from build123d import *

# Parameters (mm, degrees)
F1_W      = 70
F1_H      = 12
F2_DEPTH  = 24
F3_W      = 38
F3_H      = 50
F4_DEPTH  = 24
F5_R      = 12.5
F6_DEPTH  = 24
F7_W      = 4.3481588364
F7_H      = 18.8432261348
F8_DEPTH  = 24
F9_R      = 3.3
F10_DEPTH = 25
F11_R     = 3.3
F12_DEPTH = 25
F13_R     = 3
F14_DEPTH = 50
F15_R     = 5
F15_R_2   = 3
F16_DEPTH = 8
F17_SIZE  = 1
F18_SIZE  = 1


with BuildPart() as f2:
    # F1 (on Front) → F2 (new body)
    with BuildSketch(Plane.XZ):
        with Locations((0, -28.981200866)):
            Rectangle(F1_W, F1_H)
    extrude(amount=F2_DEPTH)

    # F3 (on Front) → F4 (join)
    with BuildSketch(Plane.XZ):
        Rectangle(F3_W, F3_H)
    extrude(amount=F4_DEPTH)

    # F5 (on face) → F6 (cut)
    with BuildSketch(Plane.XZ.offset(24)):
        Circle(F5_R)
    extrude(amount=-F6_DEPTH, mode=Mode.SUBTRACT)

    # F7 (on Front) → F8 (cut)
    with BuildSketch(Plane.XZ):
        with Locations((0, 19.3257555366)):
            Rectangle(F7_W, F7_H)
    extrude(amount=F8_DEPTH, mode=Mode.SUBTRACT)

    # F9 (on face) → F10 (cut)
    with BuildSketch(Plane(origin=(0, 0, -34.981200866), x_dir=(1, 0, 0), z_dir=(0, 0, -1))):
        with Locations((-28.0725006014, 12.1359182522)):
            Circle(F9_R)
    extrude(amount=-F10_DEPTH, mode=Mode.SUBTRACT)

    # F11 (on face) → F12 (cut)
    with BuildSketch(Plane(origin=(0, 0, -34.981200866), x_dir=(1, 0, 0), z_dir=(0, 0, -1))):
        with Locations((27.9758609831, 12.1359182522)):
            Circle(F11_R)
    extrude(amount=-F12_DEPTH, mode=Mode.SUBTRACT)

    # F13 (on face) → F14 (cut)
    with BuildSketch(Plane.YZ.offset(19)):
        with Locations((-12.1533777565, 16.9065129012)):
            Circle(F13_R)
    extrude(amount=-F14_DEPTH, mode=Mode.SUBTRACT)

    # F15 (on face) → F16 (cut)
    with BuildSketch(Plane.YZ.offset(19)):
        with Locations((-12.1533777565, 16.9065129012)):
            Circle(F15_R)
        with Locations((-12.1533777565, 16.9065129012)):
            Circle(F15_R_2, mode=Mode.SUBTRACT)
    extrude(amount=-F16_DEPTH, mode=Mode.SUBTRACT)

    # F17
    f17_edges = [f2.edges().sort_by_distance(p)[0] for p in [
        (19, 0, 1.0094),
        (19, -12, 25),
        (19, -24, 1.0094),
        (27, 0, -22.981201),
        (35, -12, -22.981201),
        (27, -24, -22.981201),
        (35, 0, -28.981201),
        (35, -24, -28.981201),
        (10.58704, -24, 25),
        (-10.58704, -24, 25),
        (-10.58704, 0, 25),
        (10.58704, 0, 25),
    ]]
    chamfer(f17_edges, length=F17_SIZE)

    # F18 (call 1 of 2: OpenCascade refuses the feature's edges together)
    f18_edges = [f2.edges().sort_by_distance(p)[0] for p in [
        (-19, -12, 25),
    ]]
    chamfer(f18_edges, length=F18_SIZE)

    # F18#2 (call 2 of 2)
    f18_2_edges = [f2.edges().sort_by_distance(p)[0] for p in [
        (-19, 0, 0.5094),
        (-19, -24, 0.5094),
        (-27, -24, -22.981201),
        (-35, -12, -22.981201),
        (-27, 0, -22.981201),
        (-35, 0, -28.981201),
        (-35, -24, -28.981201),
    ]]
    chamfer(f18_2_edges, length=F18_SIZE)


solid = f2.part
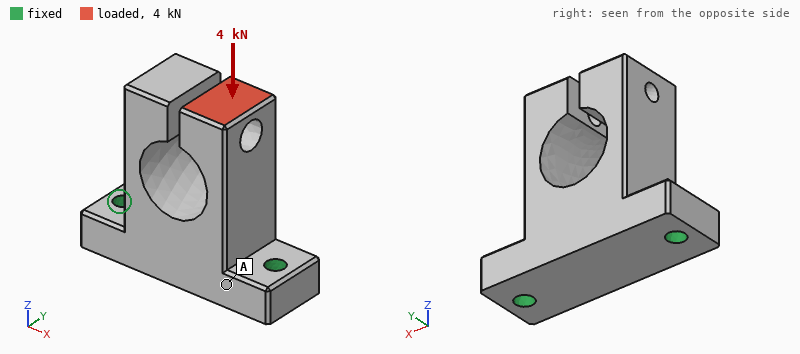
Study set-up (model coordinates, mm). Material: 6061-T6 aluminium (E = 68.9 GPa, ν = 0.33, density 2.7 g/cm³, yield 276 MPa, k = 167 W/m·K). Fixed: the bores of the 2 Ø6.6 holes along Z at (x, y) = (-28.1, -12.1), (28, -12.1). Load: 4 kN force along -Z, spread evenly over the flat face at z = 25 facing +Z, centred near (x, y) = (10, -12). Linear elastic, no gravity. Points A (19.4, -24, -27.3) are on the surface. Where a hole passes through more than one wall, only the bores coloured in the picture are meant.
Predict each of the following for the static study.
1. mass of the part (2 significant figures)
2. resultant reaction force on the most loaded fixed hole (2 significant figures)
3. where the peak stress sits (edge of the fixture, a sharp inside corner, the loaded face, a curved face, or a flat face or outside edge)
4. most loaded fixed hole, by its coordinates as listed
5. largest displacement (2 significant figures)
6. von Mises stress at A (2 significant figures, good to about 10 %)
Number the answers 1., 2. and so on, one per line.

1. 130 g
2. 3.0 kN
3. a curved face
4. (28, -12.1)
5. 0.24 mm
6. 17 MPa
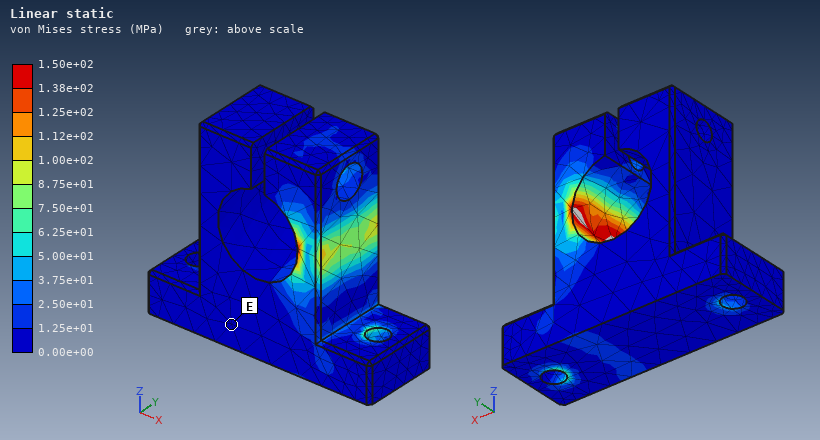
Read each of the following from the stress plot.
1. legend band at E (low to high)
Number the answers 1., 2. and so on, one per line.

1. 0.00e+00 to 1.25e+01 MPa
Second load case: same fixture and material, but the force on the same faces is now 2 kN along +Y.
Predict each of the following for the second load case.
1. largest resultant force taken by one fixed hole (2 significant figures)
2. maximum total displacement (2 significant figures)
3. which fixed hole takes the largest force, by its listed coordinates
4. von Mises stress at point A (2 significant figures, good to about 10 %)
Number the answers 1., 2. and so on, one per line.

1. 1.3 kN
2. 0.32 mm
3. (28, -12.1)
4. 100 MPa
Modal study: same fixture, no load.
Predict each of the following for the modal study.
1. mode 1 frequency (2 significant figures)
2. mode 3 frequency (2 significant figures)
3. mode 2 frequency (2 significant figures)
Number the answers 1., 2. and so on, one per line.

1. 2900 Hz
2. 3000 Hz
3. 3000 Hz
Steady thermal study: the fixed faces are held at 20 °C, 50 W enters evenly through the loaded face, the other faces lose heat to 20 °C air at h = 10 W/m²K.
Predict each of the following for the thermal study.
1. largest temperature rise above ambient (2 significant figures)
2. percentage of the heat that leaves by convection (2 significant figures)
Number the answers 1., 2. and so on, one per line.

1. 72 K
2. 4.2 %
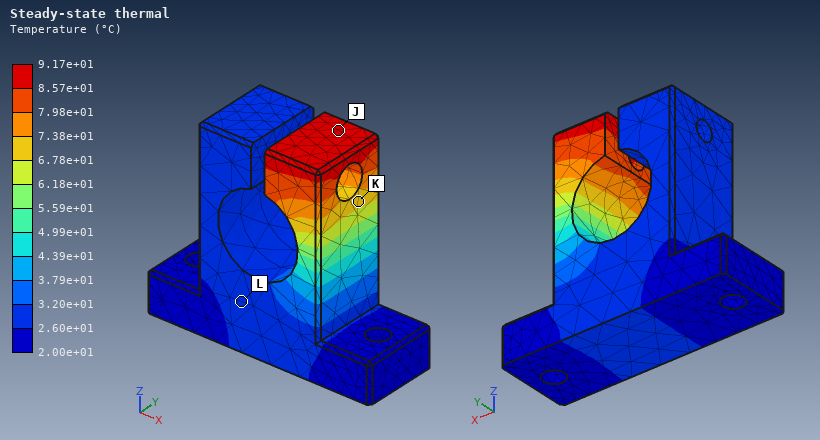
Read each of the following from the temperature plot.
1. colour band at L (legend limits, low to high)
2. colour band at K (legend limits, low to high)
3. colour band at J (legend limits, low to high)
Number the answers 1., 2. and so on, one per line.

1. 2.60e+01 to 3.20e+01 °C
2. 6.78e+01 to 7.38e+01 °C
3. 8.57e+01 to 9.17e+01 °C
